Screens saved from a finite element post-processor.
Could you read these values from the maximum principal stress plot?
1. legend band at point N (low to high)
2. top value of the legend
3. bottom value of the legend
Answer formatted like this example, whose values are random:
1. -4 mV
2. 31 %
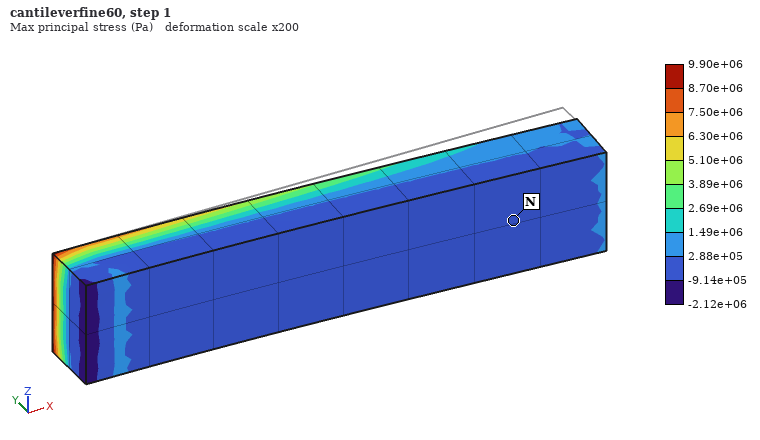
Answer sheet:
1. -9.14e+05 to 2.88e+05 Pa
2. 9.90e+06 Pa
3. -2.12e+06 Pa
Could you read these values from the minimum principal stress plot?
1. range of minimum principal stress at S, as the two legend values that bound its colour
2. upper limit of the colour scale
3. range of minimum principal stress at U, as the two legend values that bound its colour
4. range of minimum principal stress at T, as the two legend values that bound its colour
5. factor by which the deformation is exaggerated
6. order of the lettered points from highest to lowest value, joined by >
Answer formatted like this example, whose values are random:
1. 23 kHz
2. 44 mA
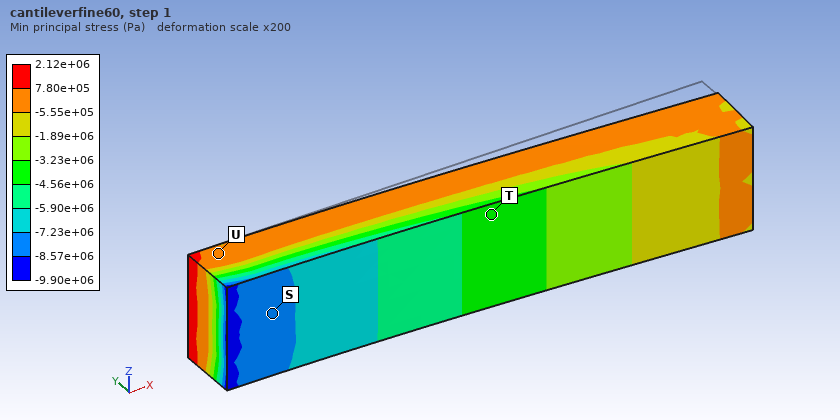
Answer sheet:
1. -8.57e+06 to -7.23e+06 Pa
2. 2.12e+06 Pa
3. -5.55e+05 to 7.80e+05 Pa
4. -4.56e+06 to -3.23e+06 Pa
5. 200
6. U > T > S
